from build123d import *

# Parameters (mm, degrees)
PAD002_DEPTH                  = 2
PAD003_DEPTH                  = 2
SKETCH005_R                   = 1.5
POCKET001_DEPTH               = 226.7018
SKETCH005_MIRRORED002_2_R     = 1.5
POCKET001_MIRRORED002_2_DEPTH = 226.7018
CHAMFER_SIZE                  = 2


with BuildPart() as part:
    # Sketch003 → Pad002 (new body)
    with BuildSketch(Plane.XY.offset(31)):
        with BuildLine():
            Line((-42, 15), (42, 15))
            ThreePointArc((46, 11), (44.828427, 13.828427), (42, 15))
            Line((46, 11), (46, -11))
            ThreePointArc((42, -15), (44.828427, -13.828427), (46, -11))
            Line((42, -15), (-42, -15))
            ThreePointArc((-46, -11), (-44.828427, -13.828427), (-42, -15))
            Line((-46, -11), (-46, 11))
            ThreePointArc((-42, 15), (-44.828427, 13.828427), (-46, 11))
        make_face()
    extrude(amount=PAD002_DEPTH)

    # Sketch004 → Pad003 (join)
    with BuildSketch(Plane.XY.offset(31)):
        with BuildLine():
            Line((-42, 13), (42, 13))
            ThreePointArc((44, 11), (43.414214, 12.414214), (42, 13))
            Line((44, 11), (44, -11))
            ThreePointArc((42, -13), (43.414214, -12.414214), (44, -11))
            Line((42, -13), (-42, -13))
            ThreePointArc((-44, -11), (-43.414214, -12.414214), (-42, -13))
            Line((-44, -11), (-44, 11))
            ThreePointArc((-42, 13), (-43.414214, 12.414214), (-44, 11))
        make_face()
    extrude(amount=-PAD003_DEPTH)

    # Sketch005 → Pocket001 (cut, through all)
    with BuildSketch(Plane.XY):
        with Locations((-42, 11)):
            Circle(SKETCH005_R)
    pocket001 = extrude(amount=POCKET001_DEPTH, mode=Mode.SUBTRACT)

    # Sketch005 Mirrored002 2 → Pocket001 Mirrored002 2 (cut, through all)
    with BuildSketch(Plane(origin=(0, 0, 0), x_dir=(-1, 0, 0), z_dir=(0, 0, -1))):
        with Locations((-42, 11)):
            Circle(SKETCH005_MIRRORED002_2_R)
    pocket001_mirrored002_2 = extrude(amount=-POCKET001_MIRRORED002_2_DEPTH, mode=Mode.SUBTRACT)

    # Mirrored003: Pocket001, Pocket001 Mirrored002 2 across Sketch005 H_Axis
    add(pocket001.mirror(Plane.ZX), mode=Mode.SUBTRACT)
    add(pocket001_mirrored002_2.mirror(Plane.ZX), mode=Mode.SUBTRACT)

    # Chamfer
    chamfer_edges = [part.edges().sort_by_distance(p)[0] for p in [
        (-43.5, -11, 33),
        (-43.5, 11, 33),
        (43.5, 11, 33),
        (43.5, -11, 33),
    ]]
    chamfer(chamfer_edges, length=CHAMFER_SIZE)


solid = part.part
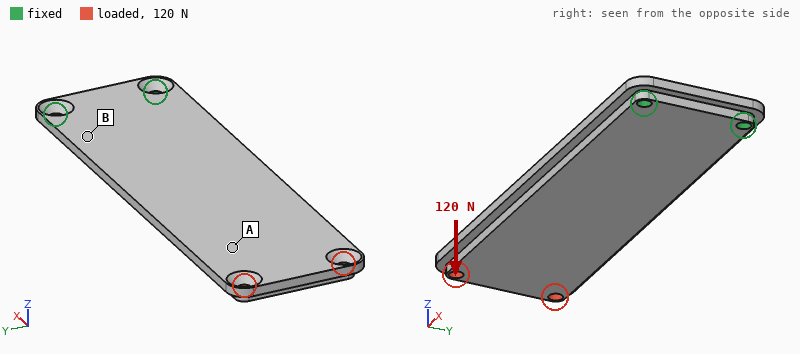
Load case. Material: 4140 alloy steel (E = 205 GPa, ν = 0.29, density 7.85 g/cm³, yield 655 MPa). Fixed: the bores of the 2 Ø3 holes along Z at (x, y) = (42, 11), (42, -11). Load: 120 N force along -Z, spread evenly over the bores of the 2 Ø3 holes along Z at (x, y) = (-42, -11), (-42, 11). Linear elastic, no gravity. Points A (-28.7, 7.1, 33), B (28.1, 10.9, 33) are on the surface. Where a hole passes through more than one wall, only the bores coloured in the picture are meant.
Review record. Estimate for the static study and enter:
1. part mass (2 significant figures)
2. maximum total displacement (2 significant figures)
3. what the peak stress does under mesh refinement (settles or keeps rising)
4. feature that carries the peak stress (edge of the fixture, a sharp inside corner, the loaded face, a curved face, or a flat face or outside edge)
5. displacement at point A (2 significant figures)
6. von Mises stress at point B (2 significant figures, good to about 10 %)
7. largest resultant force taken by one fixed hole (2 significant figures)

77 g
1.1 mm
keeps rising
edge of the fixture
0.83 mm
110 MPa
130 N
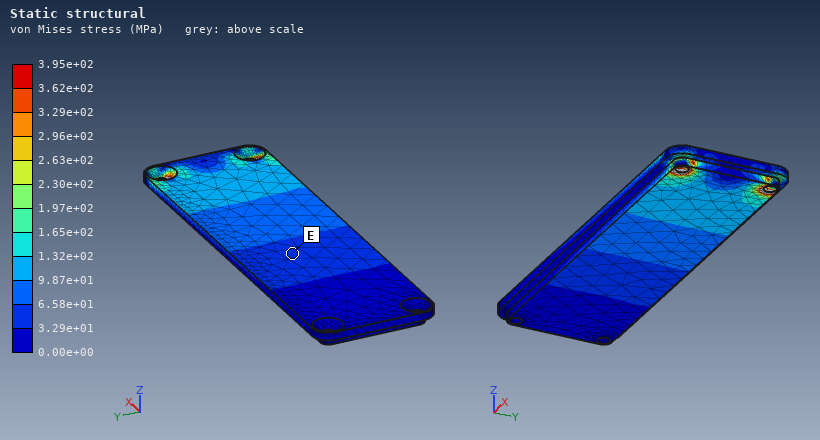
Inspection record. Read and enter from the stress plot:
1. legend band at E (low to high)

3.29e+01 to 6.58e+01 MPa
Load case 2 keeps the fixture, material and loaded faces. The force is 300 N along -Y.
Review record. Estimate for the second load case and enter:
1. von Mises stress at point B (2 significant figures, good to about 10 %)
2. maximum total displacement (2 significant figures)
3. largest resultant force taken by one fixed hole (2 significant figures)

27 MPa
54 µm
1.1 kN
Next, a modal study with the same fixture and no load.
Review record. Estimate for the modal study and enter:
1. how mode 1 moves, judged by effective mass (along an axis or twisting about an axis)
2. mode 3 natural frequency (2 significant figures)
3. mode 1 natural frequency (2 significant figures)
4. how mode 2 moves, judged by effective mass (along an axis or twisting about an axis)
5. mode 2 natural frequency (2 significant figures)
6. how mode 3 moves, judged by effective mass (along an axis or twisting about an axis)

along Z
2600 Hz
370 Hz
along Z
2400 Hz
along Y
